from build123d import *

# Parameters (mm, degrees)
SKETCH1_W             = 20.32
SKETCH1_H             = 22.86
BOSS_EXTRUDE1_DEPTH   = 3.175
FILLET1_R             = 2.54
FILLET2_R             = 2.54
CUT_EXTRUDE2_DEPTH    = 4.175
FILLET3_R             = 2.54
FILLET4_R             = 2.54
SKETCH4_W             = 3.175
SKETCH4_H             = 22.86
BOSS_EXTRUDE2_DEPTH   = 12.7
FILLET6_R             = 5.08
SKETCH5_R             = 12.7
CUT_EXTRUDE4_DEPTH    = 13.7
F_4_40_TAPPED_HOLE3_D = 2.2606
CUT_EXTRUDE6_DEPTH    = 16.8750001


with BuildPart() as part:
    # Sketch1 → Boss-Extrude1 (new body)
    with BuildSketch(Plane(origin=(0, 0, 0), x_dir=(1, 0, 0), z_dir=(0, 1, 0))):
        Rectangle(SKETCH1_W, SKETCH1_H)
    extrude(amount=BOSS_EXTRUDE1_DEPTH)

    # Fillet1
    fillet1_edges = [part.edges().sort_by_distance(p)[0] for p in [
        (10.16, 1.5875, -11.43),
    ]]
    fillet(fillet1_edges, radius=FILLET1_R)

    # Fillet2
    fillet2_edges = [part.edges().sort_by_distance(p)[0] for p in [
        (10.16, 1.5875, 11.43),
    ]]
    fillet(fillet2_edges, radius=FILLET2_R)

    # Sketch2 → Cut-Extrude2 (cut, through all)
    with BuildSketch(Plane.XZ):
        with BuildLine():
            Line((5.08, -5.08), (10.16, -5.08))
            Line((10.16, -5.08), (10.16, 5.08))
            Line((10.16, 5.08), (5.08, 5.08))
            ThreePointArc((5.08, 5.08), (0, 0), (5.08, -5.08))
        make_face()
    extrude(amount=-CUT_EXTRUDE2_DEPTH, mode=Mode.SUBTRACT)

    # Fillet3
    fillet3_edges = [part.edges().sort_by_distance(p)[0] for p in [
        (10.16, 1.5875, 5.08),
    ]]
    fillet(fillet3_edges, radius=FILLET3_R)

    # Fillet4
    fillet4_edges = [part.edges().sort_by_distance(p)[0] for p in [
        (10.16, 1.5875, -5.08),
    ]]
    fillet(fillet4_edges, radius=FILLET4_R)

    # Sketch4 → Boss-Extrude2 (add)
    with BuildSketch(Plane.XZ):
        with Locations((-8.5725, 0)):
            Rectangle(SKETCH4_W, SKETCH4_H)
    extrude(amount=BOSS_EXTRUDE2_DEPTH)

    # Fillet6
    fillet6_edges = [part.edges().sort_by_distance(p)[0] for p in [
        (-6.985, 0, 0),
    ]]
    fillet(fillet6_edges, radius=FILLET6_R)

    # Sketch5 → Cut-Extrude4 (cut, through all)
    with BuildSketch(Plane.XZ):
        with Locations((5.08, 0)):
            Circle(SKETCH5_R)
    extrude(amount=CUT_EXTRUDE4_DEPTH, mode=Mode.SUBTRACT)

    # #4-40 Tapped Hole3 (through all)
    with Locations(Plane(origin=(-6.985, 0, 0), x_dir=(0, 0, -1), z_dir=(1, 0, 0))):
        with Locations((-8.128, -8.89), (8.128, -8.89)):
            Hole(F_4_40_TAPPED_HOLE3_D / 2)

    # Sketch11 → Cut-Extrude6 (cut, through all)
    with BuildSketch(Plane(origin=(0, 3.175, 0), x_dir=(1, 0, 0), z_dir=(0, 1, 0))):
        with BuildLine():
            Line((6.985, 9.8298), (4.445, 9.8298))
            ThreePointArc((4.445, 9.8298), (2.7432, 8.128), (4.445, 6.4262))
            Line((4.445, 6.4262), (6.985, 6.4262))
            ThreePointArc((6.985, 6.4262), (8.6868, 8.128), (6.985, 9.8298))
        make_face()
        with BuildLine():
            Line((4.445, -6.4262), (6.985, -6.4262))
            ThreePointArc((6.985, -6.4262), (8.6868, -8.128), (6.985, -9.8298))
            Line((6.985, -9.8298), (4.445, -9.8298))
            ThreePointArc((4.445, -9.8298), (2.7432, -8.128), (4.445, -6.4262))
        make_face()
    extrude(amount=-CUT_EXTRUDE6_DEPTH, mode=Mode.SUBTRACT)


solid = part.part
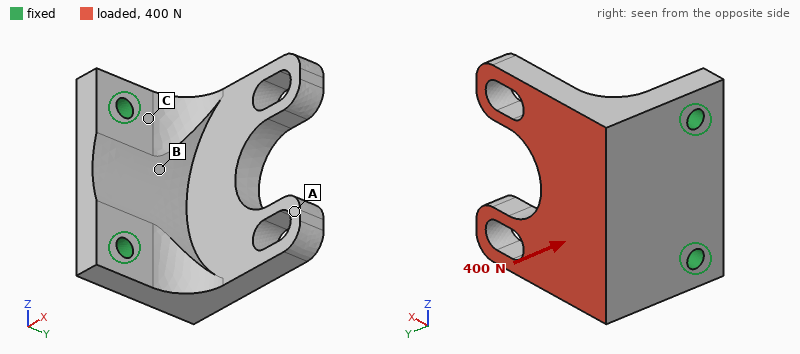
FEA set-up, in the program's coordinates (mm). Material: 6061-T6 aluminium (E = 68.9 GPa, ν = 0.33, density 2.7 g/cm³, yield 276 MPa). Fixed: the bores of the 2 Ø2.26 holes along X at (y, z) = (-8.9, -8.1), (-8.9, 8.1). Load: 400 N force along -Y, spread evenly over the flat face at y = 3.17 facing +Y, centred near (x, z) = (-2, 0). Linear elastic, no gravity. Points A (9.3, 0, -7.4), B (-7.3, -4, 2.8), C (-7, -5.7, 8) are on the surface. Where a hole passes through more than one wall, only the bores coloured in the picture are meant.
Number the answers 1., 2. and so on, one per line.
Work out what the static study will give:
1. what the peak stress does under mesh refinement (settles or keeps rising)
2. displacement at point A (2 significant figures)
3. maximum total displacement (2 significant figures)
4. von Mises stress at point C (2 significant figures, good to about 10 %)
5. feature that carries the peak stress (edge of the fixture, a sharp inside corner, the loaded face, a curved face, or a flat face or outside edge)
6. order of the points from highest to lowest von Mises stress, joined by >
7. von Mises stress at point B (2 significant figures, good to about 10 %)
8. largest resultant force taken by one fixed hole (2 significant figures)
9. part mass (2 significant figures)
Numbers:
1. keeps rising
2. 0.13 mm
3. 0.14 mm
4. 99 MPa
5. edge of the fixture
6. C > B > A
7. 46 MPa
8. 200 N
9. 5.3 g
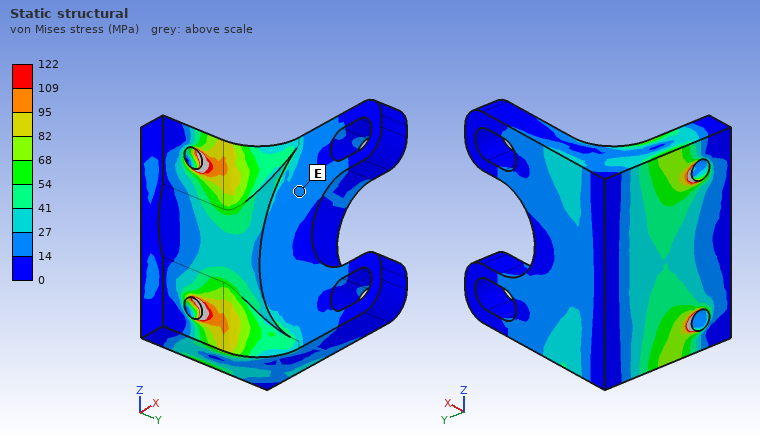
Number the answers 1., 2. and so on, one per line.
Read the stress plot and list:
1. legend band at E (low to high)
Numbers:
1. 14 to 27 MPa
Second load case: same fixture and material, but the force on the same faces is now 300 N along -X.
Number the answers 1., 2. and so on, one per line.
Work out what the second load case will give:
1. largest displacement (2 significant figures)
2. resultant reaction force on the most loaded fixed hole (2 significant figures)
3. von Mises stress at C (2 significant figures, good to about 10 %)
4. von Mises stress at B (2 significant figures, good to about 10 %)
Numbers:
1. 0.12 mm
2. 150 N
3. 94 MPa
4. 39 MPa
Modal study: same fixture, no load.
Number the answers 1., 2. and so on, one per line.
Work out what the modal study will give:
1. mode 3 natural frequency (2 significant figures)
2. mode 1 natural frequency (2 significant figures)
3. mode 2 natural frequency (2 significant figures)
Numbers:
1. 15 kHz
2. 5600 Hz
3. 9700 Hz
